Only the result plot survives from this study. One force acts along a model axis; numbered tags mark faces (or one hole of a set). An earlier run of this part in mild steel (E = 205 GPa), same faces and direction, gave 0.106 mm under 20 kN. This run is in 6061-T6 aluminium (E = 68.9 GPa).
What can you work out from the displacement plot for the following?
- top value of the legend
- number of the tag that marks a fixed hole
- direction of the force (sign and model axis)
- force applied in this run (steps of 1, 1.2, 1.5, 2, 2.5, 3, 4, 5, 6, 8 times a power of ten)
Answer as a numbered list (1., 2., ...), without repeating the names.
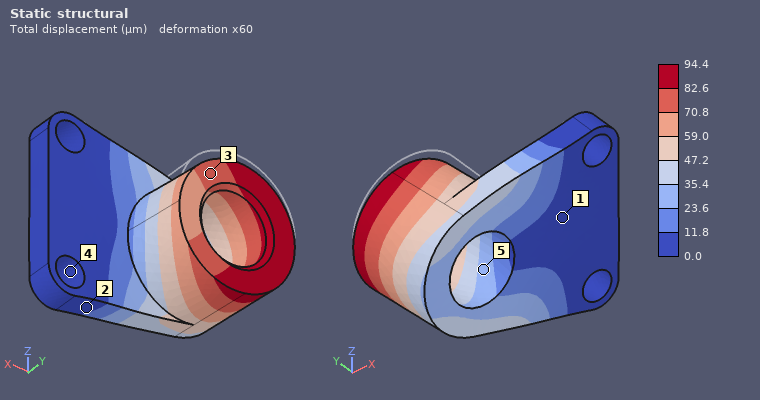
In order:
1. 94.4 µm
2. 4
3. -Z
4. 6 kN
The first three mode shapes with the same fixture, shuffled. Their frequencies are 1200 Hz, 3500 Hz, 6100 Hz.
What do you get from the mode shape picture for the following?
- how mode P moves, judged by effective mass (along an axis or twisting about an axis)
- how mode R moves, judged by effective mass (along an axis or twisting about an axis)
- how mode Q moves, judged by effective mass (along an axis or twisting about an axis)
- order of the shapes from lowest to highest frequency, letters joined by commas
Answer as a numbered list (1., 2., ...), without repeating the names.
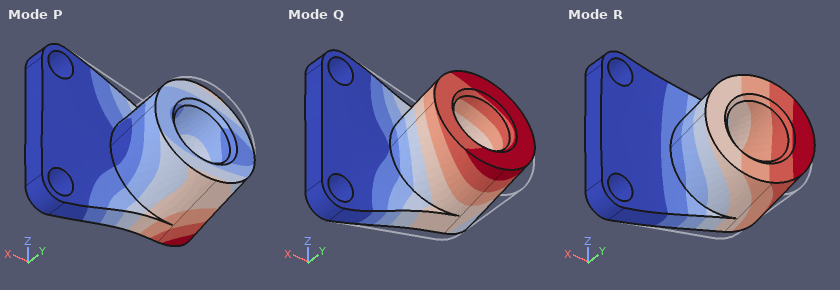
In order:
1. along Z
2. along Y
3. along Z
4. R, Q, P
